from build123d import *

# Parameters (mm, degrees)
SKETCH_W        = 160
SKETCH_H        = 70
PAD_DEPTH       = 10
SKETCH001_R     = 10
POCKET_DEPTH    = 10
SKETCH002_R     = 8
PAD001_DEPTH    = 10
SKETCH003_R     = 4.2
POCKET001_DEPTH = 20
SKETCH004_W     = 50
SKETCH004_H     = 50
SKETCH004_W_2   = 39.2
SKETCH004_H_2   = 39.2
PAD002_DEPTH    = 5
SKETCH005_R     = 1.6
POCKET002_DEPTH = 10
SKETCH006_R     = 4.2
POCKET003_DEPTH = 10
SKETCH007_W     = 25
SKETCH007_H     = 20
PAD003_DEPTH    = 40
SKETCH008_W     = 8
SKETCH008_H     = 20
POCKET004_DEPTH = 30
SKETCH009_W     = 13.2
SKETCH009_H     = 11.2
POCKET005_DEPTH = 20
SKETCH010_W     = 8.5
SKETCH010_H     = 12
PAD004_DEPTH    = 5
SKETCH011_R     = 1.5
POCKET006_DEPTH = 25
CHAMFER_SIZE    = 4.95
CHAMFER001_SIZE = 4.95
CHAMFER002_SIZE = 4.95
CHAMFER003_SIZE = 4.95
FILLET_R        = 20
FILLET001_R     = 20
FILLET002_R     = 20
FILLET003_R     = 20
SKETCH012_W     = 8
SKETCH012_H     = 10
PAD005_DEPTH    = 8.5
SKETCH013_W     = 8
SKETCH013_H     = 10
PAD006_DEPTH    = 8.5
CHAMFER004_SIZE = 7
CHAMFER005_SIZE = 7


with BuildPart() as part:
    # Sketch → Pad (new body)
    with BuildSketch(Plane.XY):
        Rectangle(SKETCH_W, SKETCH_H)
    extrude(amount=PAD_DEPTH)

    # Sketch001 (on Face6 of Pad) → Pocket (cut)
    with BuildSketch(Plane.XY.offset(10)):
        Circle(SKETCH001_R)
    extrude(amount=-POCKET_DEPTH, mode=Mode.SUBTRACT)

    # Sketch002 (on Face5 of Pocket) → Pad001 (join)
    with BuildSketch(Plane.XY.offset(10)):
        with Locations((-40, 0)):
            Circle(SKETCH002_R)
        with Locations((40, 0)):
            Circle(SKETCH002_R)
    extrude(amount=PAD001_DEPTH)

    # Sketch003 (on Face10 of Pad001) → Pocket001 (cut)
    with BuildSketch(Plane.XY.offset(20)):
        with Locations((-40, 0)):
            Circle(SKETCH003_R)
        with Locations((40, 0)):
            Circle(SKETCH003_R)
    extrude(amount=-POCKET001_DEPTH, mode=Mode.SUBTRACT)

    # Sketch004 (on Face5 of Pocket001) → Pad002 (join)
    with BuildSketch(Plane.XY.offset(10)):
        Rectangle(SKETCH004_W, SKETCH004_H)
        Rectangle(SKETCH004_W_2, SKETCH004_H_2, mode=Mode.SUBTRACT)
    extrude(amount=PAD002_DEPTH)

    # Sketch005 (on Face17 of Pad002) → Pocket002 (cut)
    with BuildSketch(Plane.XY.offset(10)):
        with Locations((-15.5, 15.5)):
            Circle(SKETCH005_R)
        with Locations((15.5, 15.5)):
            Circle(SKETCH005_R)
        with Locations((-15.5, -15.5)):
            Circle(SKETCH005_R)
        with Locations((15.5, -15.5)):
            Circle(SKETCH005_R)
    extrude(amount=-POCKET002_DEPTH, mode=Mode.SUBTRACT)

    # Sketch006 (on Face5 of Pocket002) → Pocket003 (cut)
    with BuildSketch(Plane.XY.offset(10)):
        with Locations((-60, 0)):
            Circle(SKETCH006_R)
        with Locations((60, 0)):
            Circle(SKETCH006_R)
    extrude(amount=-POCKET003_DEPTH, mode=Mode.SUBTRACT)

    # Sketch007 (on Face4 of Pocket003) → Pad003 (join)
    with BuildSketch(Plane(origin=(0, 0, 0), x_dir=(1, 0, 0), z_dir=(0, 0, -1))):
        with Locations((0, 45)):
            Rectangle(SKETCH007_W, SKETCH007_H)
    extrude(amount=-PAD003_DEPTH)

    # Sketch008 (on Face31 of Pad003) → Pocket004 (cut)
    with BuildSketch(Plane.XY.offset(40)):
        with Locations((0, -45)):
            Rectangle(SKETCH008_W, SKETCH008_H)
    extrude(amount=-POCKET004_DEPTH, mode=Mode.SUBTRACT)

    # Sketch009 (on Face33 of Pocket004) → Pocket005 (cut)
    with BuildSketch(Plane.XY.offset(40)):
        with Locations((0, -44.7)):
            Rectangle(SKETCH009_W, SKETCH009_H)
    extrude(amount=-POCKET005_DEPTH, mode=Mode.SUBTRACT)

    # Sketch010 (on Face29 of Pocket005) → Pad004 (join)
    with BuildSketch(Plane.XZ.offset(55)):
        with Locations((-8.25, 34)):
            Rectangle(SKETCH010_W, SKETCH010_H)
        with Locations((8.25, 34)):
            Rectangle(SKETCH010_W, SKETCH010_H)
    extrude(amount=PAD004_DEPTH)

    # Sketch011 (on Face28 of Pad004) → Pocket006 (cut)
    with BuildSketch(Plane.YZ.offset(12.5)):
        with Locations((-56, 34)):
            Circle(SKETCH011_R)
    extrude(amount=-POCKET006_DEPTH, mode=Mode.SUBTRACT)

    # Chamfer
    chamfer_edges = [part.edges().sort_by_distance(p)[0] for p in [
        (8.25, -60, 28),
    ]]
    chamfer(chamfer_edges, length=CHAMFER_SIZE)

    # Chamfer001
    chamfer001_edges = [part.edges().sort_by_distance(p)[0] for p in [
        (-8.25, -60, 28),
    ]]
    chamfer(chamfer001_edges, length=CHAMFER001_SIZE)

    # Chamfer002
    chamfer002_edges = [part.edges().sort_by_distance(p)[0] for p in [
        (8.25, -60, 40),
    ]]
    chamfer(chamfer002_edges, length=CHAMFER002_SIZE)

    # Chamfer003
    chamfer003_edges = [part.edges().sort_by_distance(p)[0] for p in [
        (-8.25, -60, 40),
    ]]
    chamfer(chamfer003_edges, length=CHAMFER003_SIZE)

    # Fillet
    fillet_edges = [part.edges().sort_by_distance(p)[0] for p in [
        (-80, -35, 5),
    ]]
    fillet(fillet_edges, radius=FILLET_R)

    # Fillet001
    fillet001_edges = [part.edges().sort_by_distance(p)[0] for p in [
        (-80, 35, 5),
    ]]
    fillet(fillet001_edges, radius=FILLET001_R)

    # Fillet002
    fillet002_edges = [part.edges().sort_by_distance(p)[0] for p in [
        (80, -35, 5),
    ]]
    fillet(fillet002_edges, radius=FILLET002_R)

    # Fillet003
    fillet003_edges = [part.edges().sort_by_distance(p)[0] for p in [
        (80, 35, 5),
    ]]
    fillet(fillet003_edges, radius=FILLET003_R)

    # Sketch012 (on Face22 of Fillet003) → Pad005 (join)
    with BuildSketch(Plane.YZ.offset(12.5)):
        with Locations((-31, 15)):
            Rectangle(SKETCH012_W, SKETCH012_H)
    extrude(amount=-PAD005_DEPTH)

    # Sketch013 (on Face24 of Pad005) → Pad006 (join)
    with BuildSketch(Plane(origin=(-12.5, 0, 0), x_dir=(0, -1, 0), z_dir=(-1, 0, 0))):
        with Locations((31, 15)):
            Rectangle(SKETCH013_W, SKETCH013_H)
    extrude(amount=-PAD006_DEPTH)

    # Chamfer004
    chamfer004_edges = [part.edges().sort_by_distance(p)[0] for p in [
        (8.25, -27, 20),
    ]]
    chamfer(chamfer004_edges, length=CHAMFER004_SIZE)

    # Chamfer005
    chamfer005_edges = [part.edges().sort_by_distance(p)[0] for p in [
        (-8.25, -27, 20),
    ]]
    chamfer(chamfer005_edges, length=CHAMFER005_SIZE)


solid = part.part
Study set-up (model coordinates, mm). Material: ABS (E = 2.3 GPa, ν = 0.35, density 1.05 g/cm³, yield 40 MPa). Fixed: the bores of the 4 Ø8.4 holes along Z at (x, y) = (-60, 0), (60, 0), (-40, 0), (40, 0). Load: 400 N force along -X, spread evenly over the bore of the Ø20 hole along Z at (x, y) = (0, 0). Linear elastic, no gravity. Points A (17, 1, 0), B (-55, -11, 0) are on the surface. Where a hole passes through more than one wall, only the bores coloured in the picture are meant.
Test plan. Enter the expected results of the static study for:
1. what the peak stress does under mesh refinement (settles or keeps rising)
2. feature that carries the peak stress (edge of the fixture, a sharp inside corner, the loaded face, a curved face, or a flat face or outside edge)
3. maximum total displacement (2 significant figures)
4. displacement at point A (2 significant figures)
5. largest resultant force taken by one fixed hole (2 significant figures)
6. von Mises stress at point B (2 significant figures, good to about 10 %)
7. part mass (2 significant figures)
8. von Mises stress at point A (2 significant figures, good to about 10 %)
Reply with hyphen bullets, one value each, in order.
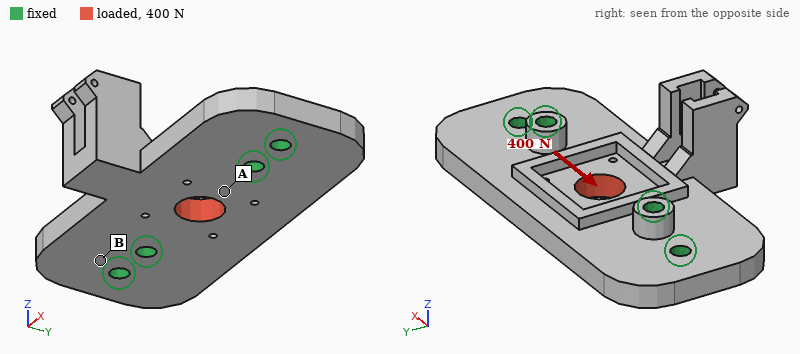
- keeps rising
- edge of the fixture
- 9.6 µm
- 6.2 µm
- 150 N
- 0.16 MPa
- 130 g
- 0.70 MPa
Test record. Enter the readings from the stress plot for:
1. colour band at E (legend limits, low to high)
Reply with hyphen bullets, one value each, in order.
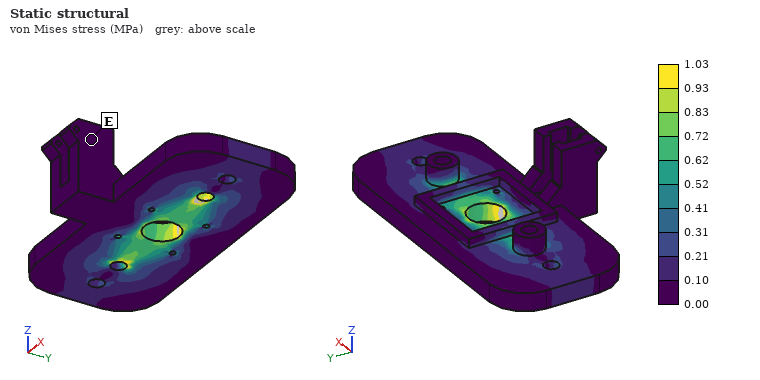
- 0.00 to 0.10 MPa
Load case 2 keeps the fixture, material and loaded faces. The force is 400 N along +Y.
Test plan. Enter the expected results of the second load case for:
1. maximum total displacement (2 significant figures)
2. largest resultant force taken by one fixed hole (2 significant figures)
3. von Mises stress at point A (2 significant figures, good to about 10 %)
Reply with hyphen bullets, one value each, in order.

- 20 µm
- 220 N
- 0.60 MPa
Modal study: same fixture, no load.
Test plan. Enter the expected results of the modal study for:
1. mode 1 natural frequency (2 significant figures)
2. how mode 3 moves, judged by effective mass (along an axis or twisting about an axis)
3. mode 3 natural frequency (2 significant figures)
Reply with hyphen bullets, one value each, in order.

- 650 Hz
- along Z
- 1600 Hz
